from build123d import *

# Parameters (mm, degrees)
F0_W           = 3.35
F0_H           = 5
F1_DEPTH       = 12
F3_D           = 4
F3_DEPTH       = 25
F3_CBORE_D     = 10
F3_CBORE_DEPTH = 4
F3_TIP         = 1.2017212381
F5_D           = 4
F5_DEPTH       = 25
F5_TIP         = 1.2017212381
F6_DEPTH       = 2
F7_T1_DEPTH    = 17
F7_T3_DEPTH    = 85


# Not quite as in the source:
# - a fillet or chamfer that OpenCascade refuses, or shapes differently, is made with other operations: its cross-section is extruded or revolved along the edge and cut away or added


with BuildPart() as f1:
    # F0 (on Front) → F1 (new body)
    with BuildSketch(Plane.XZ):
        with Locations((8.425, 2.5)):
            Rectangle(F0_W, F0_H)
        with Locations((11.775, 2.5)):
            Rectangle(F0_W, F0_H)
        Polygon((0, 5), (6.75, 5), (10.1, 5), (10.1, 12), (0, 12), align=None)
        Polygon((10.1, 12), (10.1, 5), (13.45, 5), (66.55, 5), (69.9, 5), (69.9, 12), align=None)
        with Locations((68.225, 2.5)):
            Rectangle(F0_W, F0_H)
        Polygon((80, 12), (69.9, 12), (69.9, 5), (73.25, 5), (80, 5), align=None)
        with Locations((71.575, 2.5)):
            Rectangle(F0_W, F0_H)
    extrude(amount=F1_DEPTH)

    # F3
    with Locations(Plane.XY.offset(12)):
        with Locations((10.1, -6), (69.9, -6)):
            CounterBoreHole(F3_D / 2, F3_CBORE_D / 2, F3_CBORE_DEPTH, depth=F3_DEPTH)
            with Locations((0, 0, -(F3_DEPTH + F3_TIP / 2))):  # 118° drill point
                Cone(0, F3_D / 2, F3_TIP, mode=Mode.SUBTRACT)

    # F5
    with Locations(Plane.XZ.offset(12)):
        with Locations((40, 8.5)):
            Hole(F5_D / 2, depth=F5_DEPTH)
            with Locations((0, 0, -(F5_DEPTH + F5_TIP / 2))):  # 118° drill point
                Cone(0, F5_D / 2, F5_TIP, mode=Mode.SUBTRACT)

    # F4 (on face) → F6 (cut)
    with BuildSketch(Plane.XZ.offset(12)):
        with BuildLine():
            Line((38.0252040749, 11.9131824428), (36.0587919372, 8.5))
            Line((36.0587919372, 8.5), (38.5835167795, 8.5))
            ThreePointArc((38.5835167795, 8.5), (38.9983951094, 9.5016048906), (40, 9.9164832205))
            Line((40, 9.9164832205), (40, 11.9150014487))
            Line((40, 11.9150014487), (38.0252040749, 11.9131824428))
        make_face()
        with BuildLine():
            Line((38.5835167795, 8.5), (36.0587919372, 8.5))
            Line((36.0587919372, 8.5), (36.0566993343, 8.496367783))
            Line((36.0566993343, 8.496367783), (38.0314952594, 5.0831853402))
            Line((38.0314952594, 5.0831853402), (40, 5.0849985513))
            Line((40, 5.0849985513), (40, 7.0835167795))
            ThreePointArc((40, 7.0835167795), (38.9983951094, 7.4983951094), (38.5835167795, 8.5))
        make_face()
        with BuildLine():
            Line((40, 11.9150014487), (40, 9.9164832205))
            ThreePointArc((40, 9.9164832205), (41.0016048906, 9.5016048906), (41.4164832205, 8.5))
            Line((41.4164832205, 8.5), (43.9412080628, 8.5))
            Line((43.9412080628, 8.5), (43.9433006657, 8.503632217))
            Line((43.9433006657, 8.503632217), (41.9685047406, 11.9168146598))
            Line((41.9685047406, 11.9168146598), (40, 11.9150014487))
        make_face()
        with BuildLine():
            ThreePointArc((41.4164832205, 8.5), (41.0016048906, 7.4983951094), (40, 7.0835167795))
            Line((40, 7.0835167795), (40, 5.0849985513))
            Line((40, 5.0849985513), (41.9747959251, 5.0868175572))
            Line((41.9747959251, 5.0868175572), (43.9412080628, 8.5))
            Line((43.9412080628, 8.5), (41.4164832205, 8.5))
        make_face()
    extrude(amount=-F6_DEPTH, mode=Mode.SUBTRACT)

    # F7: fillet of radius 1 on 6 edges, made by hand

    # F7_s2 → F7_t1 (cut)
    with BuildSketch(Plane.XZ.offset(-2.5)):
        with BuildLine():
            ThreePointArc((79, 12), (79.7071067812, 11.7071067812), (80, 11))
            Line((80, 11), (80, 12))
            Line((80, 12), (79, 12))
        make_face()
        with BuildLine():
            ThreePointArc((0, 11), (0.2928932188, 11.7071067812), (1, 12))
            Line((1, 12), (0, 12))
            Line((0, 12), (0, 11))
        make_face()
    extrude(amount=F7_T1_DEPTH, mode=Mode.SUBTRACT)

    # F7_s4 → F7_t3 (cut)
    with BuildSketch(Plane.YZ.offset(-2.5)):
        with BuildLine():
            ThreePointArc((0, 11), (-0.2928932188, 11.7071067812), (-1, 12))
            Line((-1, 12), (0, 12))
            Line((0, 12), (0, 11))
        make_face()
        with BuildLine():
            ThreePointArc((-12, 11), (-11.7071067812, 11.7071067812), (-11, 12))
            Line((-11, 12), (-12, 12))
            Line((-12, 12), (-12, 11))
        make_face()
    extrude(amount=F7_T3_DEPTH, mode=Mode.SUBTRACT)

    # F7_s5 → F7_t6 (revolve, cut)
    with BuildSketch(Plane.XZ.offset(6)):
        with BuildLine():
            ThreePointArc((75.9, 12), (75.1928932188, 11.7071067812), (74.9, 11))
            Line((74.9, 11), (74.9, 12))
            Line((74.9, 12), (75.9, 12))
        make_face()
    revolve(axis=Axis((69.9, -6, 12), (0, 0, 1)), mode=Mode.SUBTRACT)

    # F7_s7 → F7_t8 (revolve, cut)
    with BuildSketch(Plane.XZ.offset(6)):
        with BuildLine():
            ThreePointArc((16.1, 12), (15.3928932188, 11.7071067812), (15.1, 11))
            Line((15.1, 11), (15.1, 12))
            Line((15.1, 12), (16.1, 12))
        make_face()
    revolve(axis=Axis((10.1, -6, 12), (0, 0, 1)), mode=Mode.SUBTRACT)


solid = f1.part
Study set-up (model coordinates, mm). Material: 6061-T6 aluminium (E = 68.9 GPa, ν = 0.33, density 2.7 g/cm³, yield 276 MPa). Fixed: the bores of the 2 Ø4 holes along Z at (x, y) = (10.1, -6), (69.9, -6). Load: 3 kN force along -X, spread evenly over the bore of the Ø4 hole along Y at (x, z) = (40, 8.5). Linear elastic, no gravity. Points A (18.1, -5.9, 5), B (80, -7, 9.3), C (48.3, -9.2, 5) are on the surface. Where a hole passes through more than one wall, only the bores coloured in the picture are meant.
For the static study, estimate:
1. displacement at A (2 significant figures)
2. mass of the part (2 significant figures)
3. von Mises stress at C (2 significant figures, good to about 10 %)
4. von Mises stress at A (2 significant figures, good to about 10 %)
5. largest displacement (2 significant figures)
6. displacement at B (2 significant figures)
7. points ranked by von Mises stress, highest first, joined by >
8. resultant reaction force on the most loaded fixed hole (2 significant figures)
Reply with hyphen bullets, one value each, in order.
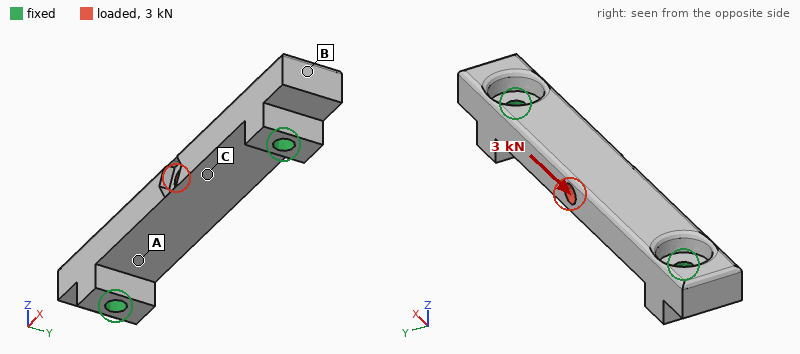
- 4.3 µm
- 17 g
- 23 MPa
- 40 MPa
- 12 µm
- 4.3 µm
- A > C > B
- 1.5 kN
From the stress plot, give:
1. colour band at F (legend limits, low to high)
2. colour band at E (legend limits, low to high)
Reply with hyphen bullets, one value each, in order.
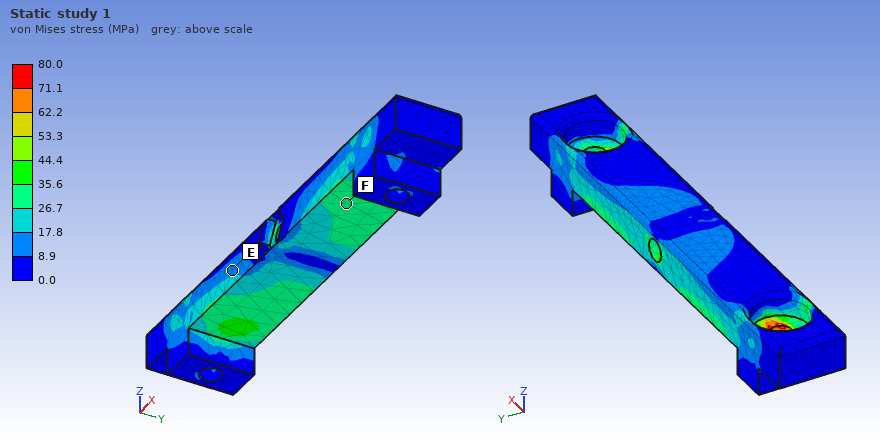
- 26.7 to 35.6 MPa
- 8.9 to 17.8 MPa
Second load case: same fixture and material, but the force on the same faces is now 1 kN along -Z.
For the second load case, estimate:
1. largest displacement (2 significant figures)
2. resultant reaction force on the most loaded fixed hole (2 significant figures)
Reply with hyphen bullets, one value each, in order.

- 80 µm
- 900 N
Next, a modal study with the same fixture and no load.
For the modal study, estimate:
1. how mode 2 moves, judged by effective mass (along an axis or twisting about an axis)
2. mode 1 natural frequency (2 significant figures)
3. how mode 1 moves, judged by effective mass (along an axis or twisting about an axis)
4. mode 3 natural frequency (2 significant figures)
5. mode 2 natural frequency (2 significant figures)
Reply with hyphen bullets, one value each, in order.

- along Y
- 8300 Hz
- along Z
- 19 kHz
- 10 kHz
